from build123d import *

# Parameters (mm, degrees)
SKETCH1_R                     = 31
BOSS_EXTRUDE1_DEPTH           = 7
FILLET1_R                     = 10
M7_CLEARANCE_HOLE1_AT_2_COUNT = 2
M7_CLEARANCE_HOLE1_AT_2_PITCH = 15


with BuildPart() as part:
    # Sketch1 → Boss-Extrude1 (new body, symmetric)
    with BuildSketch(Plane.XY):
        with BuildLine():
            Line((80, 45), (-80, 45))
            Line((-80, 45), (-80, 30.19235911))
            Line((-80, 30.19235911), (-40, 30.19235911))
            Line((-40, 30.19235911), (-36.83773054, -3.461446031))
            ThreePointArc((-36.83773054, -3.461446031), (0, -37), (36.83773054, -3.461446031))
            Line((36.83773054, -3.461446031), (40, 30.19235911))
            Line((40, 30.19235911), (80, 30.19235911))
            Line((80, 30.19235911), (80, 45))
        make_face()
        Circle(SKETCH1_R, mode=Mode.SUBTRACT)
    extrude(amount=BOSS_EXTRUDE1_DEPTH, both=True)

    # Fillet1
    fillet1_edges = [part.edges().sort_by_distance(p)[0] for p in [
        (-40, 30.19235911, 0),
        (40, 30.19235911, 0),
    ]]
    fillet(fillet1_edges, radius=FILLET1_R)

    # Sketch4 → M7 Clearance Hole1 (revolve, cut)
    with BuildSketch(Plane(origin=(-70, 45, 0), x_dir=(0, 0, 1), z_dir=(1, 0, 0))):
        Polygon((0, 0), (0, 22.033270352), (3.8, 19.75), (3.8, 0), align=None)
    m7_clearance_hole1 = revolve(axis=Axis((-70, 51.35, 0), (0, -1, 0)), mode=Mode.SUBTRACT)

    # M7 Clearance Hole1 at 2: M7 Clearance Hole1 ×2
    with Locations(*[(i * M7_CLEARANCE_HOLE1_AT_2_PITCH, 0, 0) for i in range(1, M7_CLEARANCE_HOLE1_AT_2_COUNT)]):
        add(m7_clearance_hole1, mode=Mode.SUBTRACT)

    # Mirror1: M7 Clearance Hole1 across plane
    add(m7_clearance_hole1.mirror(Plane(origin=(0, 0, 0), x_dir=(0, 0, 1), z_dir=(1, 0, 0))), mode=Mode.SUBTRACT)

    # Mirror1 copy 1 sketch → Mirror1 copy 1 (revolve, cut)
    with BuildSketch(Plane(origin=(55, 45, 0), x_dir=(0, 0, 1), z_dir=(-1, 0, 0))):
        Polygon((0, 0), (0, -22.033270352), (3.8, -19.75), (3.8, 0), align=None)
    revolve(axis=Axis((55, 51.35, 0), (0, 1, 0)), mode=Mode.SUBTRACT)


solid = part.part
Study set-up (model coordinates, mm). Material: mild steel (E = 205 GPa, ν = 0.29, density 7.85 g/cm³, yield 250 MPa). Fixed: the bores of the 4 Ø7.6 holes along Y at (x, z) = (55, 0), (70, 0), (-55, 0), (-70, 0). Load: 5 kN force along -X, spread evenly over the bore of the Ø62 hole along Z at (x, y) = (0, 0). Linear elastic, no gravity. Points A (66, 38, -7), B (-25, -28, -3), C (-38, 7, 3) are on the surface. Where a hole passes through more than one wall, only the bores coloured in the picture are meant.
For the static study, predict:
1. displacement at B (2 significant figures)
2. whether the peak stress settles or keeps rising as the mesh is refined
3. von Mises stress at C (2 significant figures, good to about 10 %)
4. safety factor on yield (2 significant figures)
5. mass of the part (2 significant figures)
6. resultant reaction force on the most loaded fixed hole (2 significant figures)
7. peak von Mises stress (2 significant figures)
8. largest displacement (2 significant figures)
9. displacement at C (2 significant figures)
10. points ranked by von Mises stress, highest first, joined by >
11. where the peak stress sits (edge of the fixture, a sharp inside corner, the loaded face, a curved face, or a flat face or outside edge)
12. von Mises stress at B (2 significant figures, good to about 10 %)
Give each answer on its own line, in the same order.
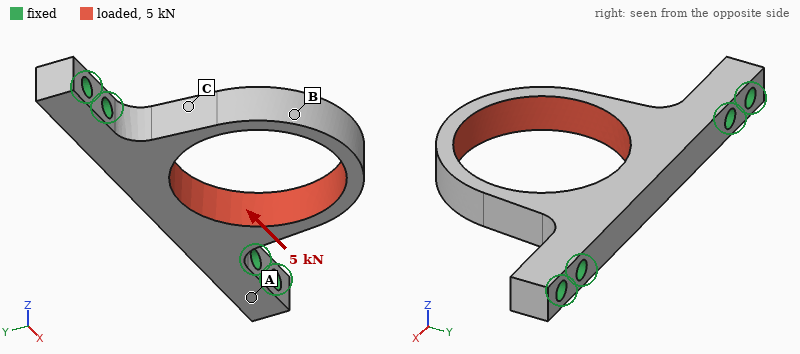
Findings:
0.12 mm
settles
130 MPa
1.9
400 g
3.0 kN
130 MPa
0.12 mm
0.023 mm
C > B > A
the loaded face
97 MPa
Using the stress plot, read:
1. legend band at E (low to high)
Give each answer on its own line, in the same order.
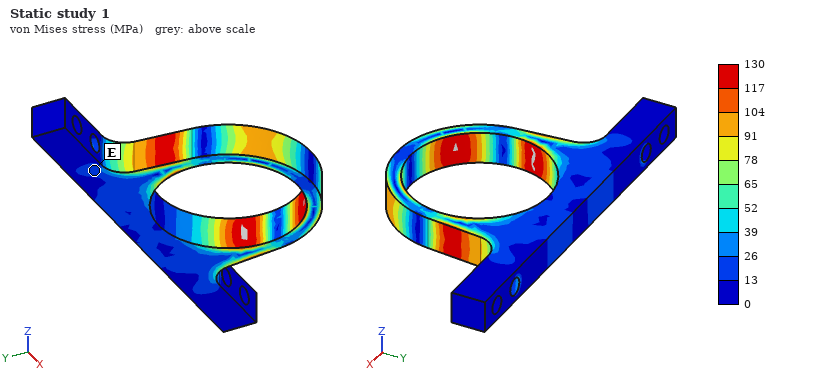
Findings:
13 to 26 MPa
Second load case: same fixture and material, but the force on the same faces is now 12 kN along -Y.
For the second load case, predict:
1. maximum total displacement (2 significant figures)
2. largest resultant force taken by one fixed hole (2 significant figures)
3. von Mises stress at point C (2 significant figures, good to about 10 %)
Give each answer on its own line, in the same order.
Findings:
42 µm
6.3 kN
97 MPa
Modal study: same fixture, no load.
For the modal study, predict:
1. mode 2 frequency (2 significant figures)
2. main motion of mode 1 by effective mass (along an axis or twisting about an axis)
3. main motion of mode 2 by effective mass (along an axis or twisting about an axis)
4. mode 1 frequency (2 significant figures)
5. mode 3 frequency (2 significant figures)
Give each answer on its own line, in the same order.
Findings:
3000 Hz
along Z
along X
1600 Hz
4000 Hz
